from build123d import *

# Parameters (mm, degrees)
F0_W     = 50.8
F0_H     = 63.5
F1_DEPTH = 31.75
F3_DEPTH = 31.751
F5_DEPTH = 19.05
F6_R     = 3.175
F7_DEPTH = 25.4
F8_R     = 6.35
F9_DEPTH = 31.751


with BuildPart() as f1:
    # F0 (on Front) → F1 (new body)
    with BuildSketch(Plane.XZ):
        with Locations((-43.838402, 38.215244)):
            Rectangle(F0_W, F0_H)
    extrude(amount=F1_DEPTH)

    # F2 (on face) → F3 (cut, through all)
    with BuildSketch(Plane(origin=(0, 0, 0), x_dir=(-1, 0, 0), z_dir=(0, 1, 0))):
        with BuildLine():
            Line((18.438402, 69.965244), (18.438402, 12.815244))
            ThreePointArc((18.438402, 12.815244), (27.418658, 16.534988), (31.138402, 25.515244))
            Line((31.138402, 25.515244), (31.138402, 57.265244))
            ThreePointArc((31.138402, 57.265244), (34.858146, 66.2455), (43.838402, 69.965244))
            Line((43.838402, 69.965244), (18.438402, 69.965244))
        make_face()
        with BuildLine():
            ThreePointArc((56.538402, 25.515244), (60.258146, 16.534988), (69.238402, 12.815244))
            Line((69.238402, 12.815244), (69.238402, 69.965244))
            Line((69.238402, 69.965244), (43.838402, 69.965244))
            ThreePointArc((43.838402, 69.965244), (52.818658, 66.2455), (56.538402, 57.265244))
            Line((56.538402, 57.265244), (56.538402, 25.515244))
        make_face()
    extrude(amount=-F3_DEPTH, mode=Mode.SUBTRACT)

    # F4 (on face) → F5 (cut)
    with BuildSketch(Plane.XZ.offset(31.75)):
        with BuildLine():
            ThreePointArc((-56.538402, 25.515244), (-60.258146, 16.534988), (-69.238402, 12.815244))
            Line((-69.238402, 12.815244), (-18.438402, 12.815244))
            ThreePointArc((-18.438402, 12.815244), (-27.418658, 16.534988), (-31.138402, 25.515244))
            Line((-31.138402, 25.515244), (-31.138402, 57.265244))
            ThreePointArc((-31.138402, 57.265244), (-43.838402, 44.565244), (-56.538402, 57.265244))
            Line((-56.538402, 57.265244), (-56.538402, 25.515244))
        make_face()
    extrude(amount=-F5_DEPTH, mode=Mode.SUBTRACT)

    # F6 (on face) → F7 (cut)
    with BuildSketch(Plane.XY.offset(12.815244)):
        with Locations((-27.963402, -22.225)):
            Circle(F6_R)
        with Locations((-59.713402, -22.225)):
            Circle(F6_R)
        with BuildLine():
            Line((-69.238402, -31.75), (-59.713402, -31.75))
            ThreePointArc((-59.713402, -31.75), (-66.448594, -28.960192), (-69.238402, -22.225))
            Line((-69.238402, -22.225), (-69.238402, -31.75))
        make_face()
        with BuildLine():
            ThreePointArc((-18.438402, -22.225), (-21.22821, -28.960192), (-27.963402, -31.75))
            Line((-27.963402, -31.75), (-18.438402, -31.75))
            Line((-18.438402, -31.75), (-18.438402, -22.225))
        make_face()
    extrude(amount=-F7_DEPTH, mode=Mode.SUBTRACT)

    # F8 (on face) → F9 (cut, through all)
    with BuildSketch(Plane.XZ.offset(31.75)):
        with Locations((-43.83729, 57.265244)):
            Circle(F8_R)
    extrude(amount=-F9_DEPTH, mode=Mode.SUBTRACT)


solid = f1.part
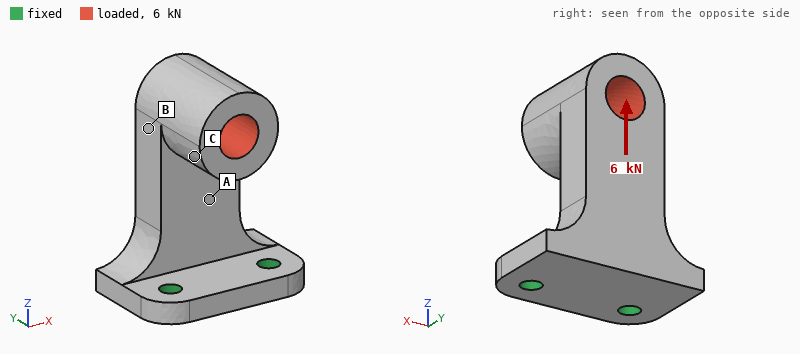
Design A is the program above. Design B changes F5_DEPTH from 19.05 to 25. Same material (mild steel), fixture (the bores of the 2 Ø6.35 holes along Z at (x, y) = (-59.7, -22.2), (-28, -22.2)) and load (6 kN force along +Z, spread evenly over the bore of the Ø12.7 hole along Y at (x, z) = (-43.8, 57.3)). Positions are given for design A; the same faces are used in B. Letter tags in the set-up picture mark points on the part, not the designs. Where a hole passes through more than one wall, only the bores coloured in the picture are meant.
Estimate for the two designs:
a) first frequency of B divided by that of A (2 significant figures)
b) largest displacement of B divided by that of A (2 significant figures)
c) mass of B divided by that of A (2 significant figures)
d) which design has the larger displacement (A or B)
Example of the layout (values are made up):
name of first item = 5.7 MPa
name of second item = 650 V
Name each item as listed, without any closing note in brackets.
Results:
first frequency of B divided by that of A = 0.65
largest displacement of B divided by that of A = 8.5
mass of B divided by that of A = 0.83
which design has the larger displacement = B
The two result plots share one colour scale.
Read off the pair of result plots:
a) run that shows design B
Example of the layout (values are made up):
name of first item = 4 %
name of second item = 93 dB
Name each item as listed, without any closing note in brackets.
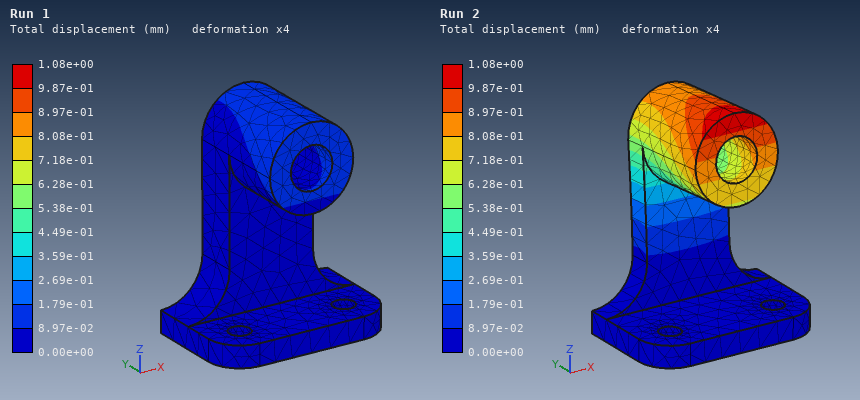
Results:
run that shows design B = Run 2
